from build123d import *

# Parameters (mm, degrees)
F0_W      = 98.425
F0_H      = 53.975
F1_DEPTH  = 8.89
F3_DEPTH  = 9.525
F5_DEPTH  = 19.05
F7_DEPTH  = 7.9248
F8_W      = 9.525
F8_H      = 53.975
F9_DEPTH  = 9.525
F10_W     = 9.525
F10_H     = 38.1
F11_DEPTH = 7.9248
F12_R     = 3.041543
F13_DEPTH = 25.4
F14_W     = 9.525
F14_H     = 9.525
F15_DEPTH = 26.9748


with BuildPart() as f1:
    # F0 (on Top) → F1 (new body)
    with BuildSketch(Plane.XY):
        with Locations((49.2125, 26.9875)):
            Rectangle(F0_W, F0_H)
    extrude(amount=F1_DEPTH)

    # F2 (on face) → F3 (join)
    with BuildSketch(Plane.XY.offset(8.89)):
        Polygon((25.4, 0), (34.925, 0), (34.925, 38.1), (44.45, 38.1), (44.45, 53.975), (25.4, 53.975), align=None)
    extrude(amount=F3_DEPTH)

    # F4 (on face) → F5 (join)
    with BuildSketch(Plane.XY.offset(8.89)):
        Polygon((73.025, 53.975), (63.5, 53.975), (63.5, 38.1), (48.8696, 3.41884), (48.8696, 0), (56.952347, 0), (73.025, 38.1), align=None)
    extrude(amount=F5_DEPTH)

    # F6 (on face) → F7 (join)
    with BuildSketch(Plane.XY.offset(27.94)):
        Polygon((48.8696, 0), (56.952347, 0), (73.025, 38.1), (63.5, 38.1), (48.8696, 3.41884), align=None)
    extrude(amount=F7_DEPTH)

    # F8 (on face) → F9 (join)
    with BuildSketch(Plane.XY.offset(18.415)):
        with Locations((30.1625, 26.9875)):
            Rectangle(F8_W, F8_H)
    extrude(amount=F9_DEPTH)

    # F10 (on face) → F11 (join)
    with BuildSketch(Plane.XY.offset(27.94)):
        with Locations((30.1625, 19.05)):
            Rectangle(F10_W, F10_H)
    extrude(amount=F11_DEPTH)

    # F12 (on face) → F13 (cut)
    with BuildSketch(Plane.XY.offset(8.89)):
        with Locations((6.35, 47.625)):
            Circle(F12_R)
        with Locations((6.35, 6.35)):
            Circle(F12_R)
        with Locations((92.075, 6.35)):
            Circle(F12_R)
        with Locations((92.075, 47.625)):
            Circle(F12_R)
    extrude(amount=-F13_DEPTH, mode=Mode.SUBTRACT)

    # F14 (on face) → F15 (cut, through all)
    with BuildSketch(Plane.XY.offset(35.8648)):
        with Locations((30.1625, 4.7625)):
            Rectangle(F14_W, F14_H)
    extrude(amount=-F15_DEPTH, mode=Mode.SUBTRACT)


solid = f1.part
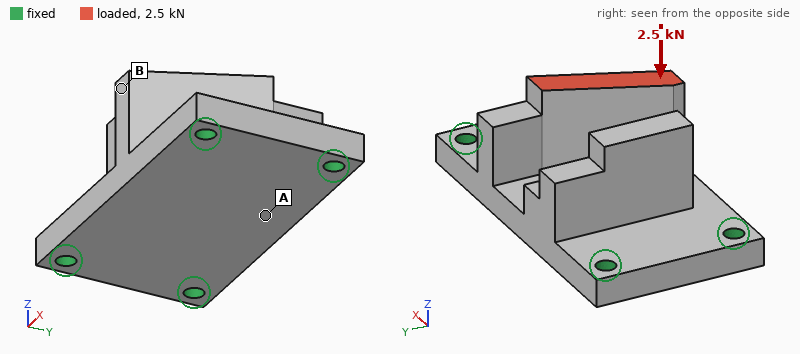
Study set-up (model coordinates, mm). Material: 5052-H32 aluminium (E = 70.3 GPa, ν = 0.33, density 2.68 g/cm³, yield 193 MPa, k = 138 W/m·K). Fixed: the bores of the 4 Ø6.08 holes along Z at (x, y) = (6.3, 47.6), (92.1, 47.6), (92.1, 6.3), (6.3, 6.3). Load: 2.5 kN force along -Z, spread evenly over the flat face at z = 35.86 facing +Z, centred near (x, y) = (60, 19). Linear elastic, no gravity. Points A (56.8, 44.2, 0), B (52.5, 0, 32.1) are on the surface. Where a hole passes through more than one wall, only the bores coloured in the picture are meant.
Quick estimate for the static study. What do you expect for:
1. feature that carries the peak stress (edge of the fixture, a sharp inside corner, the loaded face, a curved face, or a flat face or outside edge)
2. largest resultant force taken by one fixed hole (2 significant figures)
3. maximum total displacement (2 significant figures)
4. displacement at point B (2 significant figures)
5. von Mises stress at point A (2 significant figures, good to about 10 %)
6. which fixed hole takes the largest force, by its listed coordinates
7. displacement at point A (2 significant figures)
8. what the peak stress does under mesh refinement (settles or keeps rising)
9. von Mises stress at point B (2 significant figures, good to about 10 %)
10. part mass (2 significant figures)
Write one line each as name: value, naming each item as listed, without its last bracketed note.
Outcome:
feature that carries the peak stress: edge of the fixture
largest resultant force taken by one fixed hole: 1.0 kN
maximum total displacement: 60 µm
displacement at point B: 56 µm
von Mises stress at point A: 17 MPa
which fixed hole takes the largest force, by its listed coordinates: (92.1, 6.3)
displacement at point A: 25 µm
what the peak stress does under mesh refinement: keeps rising
von Mises stress at point B: 6.9 MPa
part mass: 190 g
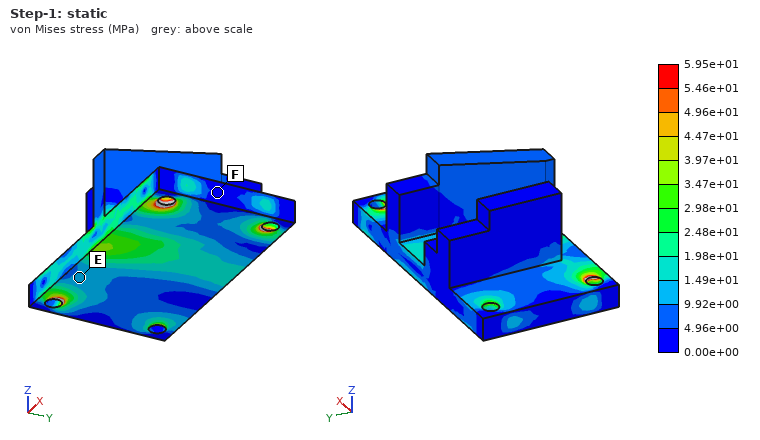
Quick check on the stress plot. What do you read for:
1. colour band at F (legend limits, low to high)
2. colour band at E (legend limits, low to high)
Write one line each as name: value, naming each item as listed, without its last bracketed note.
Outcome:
colour band at F: 0.00e+00 to 4.96e+00 MPa
colour band at E: 9.92e+00 to 1.49e+01 MPa
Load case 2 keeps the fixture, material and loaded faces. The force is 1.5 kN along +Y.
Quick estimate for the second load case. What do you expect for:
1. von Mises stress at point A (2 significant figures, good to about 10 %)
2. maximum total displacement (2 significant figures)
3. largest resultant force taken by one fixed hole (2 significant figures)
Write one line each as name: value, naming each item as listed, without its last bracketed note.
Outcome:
von Mises stress at point A: 12 MPa
maximum total displacement: 67 µm
largest resultant force taken by one fixed hole: 1.0 kN
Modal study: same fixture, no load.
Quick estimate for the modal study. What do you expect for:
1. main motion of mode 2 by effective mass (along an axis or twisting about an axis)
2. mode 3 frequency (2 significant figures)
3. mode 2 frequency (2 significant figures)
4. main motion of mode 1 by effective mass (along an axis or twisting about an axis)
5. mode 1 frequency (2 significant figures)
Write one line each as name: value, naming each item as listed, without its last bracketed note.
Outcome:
main motion of mode 2 by effective mass: along Y
mode 3 frequency: 7500 Hz
mode 2 frequency: 5500 Hz
main motion of mode 1 by effective mass: along Z
mode 1 frequency: 4000 Hz
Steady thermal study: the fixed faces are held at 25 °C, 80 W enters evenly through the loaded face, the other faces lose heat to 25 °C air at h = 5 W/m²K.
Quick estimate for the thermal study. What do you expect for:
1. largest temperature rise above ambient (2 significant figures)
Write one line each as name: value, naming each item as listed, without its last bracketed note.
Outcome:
largest temperature rise above ambient: 67 K
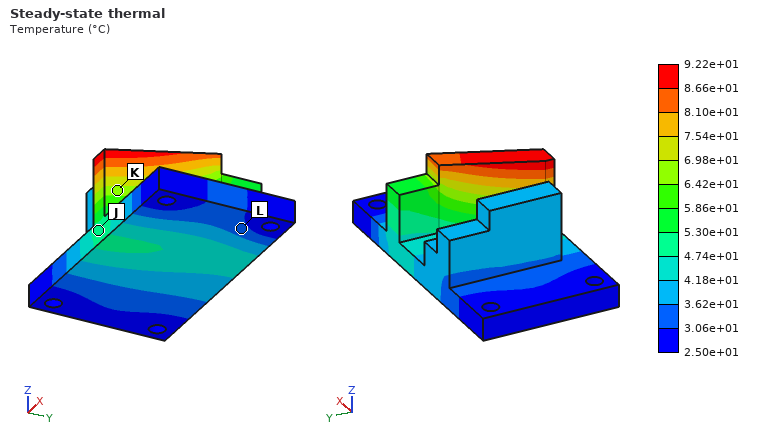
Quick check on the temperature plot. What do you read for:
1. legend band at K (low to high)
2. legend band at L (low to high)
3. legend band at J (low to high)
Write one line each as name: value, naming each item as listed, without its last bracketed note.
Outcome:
legend band at K: 6.42e+01 to 6.98e+01 °C
legend band at L: 3.06e+01 to 3.62e+01 °C
legend band at J: 4.74e+01 to 5.30e+01 °C
